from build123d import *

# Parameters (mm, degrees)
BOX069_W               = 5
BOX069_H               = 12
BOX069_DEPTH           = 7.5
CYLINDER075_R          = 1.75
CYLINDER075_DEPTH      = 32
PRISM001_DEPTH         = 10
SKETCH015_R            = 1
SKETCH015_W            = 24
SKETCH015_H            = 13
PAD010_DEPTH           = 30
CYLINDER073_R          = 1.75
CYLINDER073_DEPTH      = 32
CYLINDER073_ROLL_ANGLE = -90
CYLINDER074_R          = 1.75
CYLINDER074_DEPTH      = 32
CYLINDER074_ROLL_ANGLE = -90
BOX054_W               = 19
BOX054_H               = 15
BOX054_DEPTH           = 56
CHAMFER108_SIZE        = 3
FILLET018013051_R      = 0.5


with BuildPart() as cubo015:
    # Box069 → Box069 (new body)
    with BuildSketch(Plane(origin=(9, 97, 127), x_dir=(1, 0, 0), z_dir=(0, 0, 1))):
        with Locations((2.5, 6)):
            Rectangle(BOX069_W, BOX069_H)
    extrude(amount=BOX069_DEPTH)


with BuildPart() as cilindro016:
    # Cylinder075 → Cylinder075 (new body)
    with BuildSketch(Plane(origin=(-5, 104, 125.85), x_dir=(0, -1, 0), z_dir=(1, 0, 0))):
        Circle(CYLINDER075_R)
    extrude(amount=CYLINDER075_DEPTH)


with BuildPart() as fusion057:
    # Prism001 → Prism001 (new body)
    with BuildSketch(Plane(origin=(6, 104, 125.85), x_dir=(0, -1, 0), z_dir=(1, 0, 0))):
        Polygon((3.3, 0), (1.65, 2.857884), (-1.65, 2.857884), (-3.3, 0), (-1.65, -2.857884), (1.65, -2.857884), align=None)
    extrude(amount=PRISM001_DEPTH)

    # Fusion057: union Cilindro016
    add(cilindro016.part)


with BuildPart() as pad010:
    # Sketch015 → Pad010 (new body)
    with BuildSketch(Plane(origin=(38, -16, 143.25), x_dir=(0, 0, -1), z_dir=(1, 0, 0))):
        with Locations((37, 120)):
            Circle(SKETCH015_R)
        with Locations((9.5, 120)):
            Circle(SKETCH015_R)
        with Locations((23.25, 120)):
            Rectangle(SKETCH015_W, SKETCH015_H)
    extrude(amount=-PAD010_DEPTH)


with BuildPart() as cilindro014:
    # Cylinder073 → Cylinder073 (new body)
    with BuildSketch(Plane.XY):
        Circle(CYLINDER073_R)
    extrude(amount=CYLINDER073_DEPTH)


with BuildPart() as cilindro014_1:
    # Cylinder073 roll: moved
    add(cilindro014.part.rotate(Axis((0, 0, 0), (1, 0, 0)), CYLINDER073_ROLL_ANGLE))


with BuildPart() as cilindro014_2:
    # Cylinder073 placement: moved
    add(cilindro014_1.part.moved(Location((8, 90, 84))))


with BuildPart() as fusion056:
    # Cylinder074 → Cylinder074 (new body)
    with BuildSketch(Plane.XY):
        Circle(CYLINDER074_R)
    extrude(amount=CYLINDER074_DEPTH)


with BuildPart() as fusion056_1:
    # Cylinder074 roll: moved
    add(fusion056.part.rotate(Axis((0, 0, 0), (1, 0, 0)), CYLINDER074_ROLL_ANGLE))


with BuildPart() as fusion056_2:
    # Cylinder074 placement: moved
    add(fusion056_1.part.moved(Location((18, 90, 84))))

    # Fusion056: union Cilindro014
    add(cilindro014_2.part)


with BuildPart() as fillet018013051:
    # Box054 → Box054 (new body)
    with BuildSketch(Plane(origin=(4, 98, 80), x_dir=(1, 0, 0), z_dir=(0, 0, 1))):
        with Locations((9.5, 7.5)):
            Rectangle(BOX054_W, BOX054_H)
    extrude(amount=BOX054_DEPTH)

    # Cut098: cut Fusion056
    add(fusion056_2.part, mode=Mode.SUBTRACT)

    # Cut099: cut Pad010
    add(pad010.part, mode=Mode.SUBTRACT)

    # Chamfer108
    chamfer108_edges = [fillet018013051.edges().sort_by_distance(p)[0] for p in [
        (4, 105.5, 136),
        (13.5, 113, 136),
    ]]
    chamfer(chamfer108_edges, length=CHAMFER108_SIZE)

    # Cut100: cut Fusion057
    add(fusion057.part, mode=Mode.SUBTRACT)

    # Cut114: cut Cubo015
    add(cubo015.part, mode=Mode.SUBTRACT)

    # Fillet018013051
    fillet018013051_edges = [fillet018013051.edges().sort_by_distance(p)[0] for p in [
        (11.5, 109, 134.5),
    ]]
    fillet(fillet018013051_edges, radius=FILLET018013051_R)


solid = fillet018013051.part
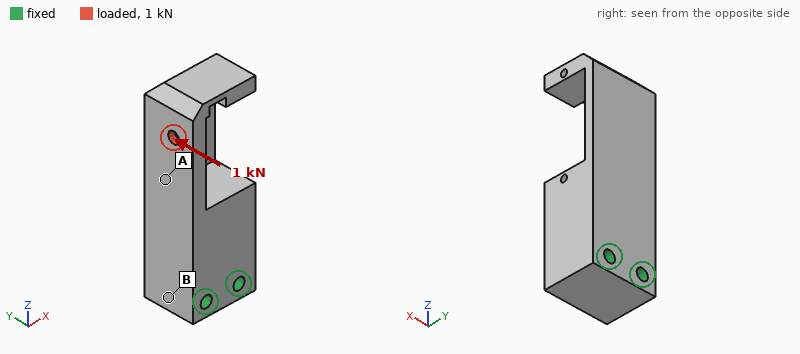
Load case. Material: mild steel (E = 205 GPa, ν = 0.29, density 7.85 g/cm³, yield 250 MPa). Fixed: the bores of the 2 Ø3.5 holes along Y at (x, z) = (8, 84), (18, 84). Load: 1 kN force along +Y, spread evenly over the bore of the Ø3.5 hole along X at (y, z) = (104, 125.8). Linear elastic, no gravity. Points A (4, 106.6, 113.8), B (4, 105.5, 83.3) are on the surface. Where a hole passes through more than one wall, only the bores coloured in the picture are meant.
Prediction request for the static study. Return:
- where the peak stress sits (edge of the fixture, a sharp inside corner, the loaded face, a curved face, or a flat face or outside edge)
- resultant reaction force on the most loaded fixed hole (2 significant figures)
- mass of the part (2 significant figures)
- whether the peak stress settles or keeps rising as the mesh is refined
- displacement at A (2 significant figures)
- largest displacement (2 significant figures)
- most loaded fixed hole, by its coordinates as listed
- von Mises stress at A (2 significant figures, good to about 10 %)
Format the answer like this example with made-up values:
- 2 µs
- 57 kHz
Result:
- a sharp inside corner
- 820 N
- 84 g
- keeps rising
- 21 µm
- 61 µm
- (8, 84)
- 55 MPa
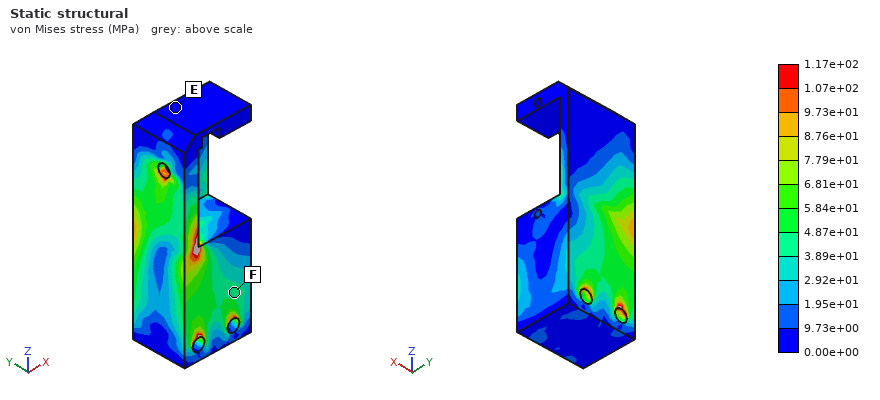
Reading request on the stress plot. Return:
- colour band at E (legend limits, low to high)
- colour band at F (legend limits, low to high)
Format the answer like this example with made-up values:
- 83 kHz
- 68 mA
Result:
- 0.00e+00 to 9.73e+00 MPa
- 3.89e+01 to 4.87e+01 MPa
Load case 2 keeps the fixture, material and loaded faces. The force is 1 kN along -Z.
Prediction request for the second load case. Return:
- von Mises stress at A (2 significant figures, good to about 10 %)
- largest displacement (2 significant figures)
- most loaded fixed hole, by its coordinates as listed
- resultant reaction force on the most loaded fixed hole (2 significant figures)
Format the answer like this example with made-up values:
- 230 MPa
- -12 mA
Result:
- 20 MPa
- 13 µm
- (8, 84)
- 1.2 kN
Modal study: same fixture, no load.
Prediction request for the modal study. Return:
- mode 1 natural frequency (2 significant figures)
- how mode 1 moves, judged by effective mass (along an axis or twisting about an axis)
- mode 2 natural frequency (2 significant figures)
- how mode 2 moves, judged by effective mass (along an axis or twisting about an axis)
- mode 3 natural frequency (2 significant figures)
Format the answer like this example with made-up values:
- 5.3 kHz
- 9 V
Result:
- 4100 Hz
- along Y
- 5200 Hz
- along X
- 9200 Hz
